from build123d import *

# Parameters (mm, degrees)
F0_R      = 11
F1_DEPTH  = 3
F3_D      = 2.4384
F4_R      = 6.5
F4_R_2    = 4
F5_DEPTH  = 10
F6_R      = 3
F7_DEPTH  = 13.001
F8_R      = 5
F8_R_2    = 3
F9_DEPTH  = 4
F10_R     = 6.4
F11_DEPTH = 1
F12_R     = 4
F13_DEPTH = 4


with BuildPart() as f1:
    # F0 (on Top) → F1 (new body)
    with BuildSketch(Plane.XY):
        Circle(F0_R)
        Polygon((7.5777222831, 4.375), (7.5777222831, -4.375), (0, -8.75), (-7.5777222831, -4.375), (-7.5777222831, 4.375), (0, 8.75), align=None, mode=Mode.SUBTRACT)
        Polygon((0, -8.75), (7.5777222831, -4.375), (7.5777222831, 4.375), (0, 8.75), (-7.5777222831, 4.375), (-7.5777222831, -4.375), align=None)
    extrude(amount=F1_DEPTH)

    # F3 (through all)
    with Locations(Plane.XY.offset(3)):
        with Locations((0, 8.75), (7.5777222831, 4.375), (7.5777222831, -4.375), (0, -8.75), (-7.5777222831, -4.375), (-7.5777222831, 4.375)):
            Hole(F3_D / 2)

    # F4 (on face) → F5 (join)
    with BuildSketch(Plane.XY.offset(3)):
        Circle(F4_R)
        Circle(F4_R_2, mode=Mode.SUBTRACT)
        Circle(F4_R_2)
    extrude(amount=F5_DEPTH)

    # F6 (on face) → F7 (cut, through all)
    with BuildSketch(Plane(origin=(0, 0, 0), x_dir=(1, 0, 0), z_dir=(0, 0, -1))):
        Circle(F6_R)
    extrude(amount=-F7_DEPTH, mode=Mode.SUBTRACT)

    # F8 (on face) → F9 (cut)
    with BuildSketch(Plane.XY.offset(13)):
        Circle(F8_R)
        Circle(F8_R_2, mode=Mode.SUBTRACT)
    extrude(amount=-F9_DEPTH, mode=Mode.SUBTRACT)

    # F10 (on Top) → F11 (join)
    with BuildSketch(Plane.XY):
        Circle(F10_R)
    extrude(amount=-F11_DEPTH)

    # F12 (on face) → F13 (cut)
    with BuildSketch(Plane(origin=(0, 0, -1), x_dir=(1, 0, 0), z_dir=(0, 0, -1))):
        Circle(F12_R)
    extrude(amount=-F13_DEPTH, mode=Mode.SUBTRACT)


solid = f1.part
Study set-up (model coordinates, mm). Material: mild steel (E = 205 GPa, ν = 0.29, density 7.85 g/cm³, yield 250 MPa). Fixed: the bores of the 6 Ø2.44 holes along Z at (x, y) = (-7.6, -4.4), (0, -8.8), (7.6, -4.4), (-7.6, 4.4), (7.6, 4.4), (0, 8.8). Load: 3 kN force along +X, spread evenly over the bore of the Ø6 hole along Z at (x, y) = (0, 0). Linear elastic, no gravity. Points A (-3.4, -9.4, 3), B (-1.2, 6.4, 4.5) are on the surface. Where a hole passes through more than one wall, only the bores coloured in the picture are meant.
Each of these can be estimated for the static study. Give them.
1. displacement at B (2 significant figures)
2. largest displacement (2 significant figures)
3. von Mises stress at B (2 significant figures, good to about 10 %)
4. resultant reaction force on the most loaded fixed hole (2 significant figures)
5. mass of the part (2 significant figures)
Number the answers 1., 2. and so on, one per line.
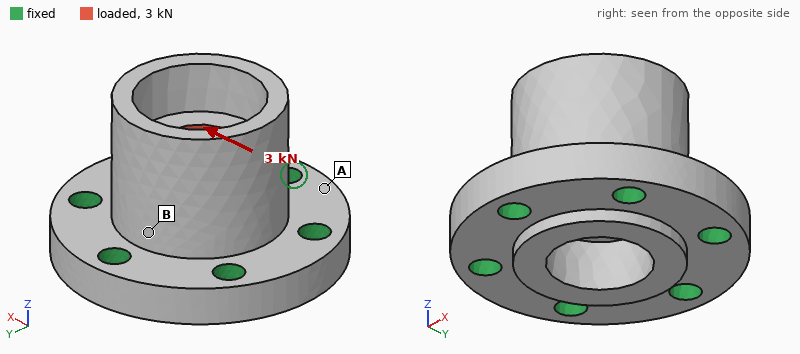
1. 1.6 µm
2. 4.5 µm
3. 39 MPa
4. 780 N
5. 14 g
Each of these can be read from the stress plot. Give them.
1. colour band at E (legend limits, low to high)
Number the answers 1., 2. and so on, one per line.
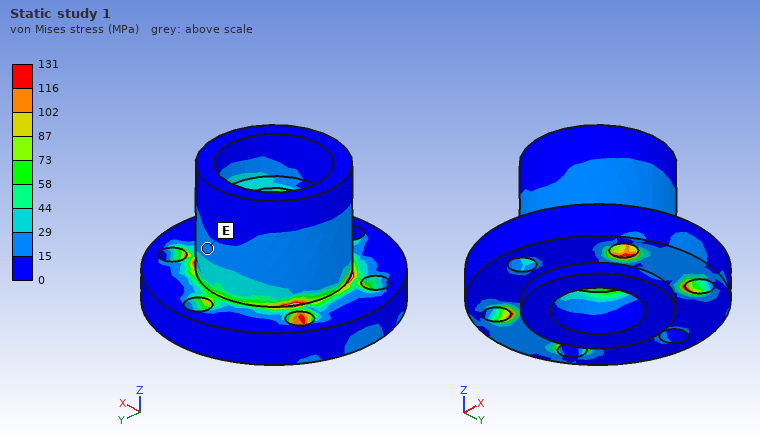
1. 15 to 29 MPa
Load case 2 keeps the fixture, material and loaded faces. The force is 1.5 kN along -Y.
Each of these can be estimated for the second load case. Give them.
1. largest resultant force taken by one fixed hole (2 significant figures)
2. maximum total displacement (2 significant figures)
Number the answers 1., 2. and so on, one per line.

1. 440 N
2. 2.3 µm
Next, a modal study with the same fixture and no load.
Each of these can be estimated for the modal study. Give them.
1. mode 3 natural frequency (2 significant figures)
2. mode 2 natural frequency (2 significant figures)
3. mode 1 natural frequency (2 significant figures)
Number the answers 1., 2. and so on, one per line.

1. 60 kHz
2. 46 kHz
3. 45 kHz
